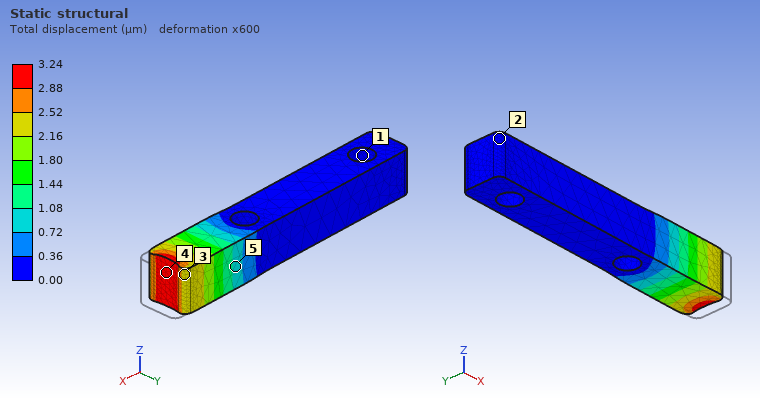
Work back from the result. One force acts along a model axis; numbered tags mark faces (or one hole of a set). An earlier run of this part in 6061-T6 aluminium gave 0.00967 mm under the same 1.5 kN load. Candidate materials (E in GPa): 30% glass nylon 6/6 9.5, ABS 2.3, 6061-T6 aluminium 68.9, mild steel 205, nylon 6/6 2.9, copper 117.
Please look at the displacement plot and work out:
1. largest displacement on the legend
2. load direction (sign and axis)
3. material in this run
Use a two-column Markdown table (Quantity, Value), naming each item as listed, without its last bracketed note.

| Quantity | Value |
|---|---|
| largest displacement on the legend | 3.24 µm |
| load direction | -X |
| material in this run | mild steel |
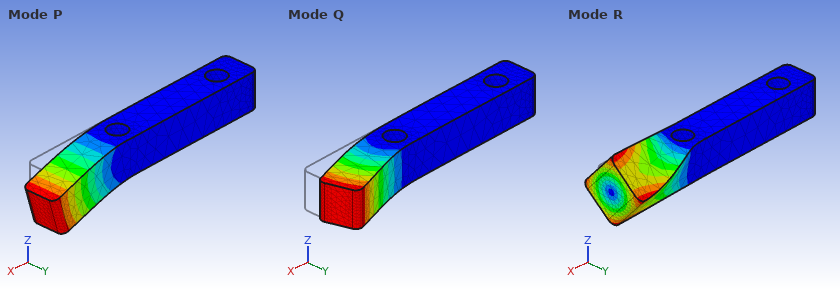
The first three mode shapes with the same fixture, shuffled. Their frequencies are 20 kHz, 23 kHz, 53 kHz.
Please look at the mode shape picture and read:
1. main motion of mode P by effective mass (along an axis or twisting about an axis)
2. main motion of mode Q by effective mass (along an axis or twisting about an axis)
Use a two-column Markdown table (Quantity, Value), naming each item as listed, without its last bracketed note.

| Quantity | Value |
|---|---|
| main motion of mode P by effective mass | along Z |
| main motion of mode Q by effective mass | along Y |
